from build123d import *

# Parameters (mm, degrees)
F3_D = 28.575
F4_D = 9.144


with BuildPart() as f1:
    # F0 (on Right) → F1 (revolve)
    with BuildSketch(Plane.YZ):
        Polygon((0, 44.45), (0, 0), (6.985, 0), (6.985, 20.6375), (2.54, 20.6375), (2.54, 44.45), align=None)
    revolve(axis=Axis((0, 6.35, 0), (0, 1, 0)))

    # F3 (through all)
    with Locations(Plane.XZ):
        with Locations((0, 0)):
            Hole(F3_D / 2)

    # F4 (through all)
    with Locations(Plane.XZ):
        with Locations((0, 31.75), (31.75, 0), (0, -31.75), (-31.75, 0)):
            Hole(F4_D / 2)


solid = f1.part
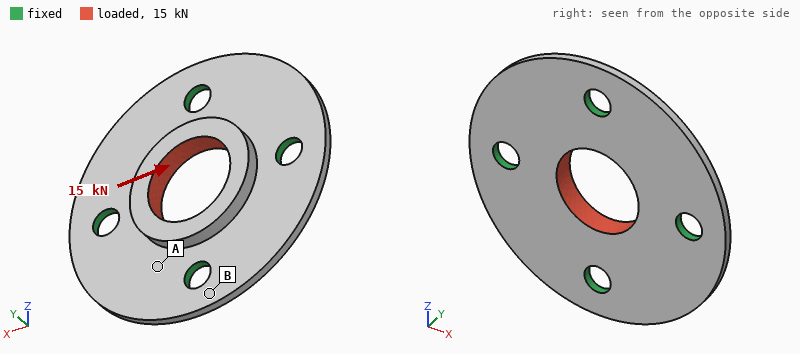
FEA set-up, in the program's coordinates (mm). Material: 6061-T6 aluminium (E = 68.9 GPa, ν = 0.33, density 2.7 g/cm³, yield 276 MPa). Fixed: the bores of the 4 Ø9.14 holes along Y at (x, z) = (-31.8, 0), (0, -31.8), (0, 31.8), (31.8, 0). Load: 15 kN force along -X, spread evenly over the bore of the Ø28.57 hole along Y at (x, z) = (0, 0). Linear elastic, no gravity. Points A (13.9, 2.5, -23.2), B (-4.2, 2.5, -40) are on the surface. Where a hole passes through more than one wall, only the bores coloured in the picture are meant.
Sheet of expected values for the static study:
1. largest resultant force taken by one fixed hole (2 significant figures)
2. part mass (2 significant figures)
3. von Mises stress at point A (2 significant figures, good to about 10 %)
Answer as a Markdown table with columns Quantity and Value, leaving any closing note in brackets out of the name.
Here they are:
| Quantity | Value |
|---|---|
| largest resultant force taken by one fixed hole | 4.5 kN |
| part mass | 45 g |
| von Mises stress at point A | 31 MPa |
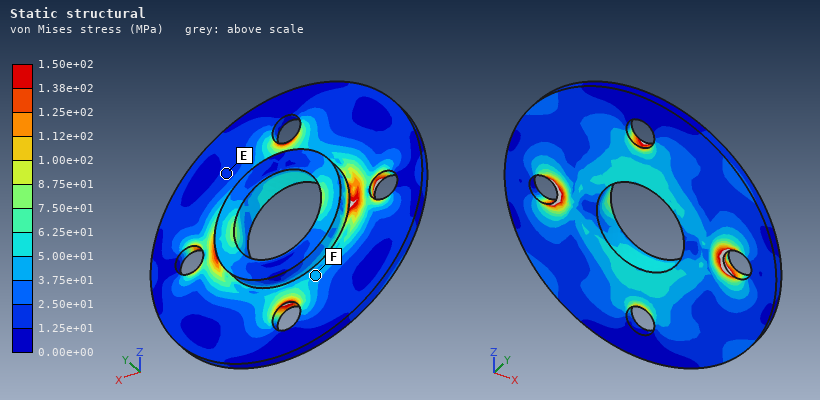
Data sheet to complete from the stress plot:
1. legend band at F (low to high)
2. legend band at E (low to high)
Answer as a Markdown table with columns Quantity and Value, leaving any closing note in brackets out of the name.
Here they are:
| Quantity | Value |
|---|---|
| legend band at F | 3.75e+01 to 5.00e+01 MPa |
| legend band at E | 1.25e+01 to 2.50e+01 MPa |
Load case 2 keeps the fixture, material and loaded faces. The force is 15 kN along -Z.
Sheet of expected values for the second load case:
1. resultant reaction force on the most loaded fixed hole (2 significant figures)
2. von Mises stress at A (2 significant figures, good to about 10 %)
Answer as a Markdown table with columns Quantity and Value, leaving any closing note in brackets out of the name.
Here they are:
| Quantity | Value |
|---|---|
| resultant reaction force on the most loaded fixed hole | 4.5 kN |
| von Mises stress at A | 45 MPa |
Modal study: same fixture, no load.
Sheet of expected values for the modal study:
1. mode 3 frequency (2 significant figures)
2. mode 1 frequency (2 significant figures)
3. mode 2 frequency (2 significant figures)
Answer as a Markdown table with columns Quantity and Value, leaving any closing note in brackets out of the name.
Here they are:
| Quantity | Value |
|---|---|
| mode 3 frequency | 5300 Hz |
| mode 1 frequency | 5200 Hz |
| mode 2 frequency | 5300 Hz |
